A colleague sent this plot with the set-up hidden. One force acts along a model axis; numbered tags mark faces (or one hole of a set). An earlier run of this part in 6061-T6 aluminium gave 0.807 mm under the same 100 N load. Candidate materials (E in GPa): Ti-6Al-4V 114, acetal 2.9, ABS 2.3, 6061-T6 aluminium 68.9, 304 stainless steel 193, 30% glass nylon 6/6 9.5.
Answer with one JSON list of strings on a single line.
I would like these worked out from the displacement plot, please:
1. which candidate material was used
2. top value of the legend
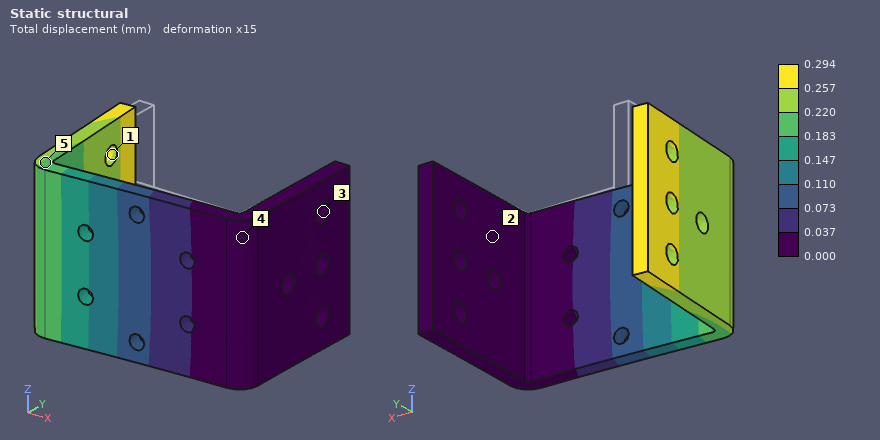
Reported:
["304 stainless steel", "0.294 mm"]
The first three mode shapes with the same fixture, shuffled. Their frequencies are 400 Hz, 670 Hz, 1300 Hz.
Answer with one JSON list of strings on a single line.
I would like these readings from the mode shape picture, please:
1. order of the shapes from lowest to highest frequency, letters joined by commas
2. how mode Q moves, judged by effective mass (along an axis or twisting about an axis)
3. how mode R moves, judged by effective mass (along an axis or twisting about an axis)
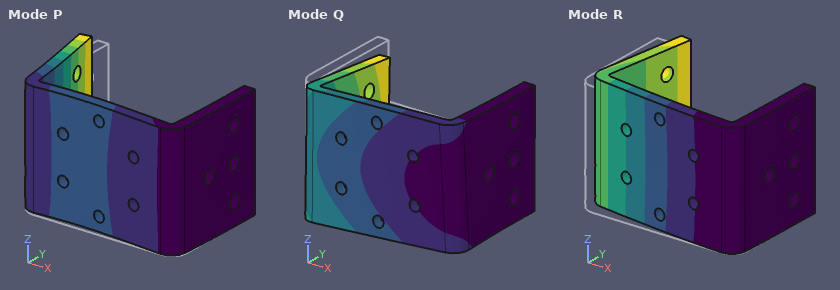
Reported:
["R, Q, P", "along Z", "along Y"]
